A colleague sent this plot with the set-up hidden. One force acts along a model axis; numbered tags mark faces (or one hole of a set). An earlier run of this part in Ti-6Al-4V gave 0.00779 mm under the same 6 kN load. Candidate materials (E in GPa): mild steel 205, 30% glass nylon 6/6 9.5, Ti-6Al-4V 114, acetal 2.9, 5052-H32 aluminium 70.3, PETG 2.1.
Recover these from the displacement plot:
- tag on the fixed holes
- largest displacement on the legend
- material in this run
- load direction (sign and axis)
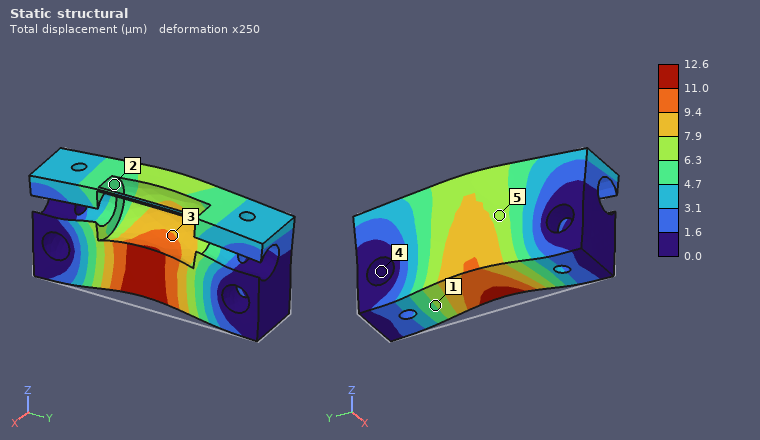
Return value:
4
12.6 µm
5052-H32 aluminium
+Z
